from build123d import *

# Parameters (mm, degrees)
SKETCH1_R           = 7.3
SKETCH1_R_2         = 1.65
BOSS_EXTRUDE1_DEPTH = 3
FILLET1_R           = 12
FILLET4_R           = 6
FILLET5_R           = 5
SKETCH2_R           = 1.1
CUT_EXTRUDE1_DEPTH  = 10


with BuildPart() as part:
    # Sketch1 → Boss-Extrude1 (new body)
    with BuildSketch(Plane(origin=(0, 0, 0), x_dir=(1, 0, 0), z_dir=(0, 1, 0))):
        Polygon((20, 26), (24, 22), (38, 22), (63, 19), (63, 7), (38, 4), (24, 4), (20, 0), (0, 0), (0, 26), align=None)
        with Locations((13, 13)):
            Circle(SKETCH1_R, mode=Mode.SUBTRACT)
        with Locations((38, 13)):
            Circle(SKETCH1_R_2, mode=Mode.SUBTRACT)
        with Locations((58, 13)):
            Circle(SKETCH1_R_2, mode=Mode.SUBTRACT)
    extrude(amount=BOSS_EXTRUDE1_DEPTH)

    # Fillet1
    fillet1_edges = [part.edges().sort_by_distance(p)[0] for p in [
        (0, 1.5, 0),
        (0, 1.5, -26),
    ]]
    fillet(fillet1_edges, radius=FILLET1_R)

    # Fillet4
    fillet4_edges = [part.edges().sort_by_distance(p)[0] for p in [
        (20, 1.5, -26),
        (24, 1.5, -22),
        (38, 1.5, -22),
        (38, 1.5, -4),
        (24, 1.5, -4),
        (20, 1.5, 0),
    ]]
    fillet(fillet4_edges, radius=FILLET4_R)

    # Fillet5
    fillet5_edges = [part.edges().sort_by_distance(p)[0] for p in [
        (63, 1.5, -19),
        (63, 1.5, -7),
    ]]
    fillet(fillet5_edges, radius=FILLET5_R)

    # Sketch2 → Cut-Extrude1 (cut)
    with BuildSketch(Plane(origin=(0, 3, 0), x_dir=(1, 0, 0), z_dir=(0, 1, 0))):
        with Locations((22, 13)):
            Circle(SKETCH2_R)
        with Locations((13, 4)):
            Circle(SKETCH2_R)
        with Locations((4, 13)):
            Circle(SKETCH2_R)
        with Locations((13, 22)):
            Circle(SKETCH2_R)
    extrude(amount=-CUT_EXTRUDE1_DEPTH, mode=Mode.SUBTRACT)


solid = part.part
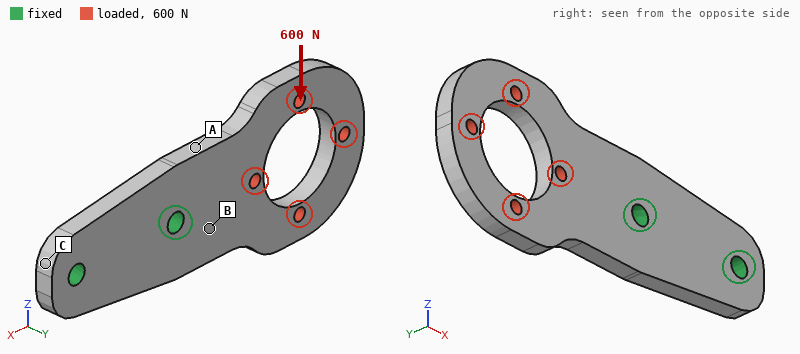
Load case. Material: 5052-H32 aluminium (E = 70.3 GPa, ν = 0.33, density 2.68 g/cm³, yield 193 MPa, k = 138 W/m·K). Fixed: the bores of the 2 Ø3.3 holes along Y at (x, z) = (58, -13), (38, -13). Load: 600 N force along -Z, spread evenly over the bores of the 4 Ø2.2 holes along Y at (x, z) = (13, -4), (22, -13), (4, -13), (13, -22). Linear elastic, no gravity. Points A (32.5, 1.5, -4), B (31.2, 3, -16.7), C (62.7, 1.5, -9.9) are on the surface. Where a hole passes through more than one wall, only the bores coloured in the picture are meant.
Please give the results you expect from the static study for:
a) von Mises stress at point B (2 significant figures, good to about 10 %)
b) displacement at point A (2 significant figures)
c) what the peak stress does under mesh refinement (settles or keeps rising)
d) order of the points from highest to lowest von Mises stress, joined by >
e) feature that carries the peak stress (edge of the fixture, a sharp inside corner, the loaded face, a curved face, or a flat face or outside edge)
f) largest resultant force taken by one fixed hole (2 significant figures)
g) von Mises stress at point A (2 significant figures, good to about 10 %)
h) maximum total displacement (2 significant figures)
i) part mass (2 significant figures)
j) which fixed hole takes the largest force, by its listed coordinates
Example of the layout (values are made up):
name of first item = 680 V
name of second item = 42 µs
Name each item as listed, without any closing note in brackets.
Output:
von Mises stress at point B = 33 MPa
displacement at point A = 0.024 mm
what the peak stress does under mesh refinement = keeps rising
order of the points from highest to lowest von Mises stress, joined by > = A > B > C
feature that carries the peak stress = edge of the fixture
largest resultant force taken by one fixed hole = 1.2 kN
von Mises stress at point A = 77 MPa
maximum total displacement = 0.15 mm
part mass = 7.8 g
which fixed hole takes the largest force, by its listed coordinates = (38, -13)
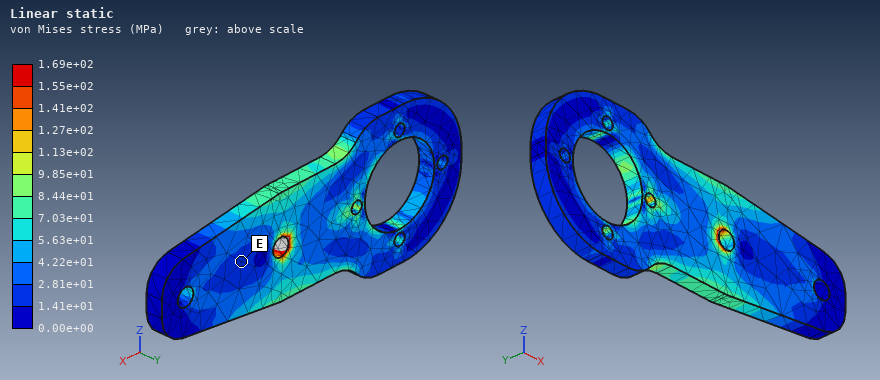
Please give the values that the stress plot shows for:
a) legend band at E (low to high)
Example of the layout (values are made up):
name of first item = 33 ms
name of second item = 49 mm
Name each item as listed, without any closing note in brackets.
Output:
legend band at E = 1.41e+01 to 2.81e+01 MPa
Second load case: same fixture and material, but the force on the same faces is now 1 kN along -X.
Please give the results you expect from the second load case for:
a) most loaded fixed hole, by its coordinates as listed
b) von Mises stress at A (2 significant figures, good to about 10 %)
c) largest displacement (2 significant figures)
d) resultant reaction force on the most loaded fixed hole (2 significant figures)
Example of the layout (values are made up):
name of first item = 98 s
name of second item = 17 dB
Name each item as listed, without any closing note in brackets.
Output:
most loaded fixed hole, by its coordinates as listed = (38, -13)
von Mises stress at A = 15 MPa
largest displacement = 22 µm
resultant reaction force on the most loaded fixed hole = 850 N
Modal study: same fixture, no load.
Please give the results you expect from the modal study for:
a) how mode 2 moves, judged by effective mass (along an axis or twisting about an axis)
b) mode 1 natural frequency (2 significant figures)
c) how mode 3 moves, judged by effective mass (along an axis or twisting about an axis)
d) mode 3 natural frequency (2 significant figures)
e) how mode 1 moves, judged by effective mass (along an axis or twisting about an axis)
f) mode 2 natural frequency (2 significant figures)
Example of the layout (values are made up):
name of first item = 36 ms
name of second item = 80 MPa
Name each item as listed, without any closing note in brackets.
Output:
how mode 2 moves, judged by effective mass = twisting about X
mode 1 natural frequency = 1900 Hz
how mode 3 moves, judged by effective mass = along Z
mode 3 natural frequency = 6400 Hz
how mode 1 moves, judged by effective mass = along Y
mode 2 natural frequency = 4600 Hz
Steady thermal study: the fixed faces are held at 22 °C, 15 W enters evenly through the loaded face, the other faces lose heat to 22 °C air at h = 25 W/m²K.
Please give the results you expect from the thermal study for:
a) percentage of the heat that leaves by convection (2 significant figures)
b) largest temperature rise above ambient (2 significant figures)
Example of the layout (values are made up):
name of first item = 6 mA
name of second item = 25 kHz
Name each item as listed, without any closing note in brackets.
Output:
percentage of the heat that leaves by convection = 10 %
largest temperature rise above ambient = 64 K
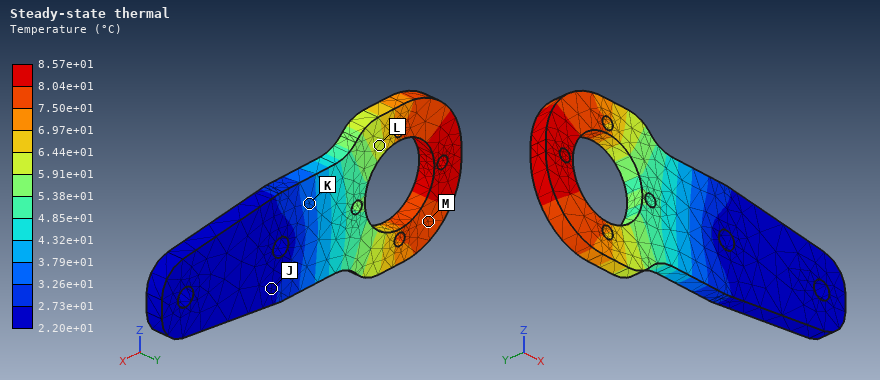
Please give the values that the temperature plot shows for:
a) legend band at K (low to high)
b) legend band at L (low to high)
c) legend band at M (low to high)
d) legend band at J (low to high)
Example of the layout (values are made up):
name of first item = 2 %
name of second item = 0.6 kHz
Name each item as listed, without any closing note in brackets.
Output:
legend band at K = 3.26e+01 to 3.79e+01 °C
legend band at L = 5.91e+01 to 6.44e+01 °C
legend band at M = 7.50e+01 to 8.04e+01 °C
legend band at J = 2.20e+01 to 2.73e+01 °C
